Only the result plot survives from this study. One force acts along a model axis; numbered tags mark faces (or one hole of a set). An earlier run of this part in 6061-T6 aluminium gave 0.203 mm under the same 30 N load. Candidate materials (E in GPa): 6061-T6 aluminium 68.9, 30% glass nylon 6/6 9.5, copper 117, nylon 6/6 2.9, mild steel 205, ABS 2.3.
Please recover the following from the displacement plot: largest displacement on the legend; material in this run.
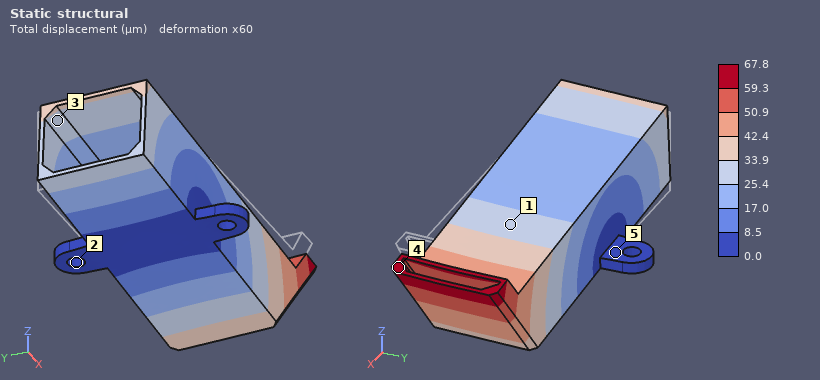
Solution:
67.8 µm
mild steel
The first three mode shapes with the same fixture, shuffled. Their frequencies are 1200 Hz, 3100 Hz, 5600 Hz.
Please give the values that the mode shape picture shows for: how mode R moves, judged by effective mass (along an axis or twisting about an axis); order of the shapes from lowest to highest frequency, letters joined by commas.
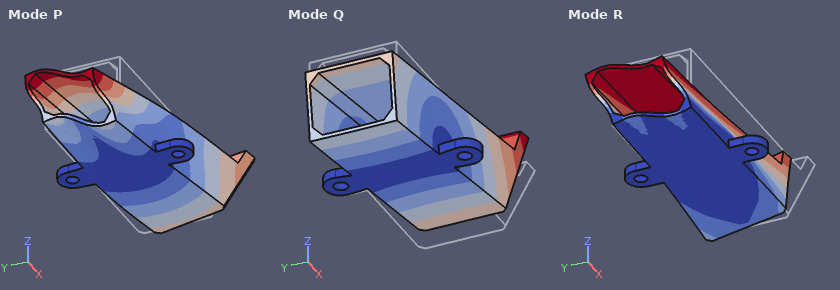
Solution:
along Y
Q, R, P
